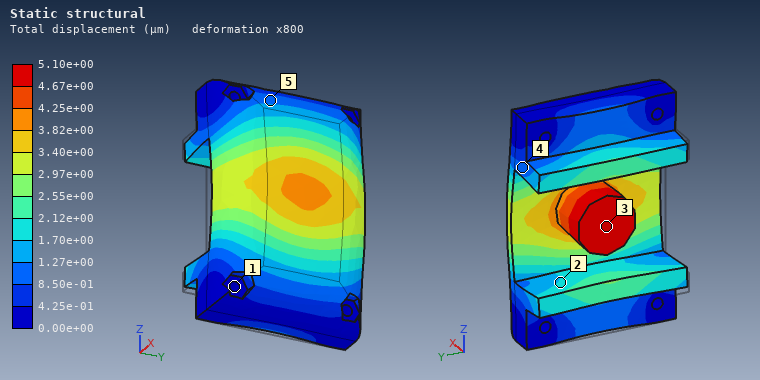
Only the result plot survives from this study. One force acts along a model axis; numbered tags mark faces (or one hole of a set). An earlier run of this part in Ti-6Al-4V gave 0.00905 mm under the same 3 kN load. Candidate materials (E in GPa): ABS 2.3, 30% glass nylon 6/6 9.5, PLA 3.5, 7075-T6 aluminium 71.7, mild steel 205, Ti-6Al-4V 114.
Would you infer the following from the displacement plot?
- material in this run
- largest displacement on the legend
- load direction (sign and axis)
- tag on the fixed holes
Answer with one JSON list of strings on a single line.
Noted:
["mild steel", "5.10e+00 µm", "+X", "1"]
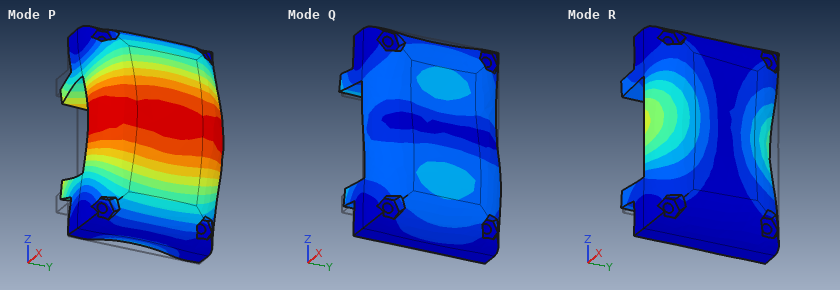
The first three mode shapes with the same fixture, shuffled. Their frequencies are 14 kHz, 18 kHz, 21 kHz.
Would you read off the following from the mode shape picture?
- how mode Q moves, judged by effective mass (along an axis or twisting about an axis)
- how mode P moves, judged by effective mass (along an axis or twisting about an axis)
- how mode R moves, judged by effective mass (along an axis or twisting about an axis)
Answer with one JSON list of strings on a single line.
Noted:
["along Z", "along X", "along Y"]
